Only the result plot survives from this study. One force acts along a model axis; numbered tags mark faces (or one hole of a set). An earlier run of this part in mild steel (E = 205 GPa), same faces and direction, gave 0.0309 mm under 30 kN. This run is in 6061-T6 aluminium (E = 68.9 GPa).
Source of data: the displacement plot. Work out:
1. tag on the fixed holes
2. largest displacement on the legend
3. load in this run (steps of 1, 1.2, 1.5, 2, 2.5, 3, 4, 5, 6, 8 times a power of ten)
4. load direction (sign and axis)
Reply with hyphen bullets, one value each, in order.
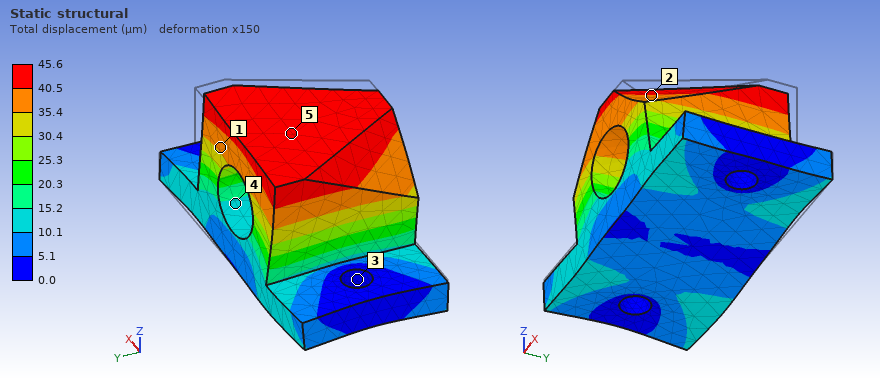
- 3
- 45.6 µm
- 15 kN
- -X
